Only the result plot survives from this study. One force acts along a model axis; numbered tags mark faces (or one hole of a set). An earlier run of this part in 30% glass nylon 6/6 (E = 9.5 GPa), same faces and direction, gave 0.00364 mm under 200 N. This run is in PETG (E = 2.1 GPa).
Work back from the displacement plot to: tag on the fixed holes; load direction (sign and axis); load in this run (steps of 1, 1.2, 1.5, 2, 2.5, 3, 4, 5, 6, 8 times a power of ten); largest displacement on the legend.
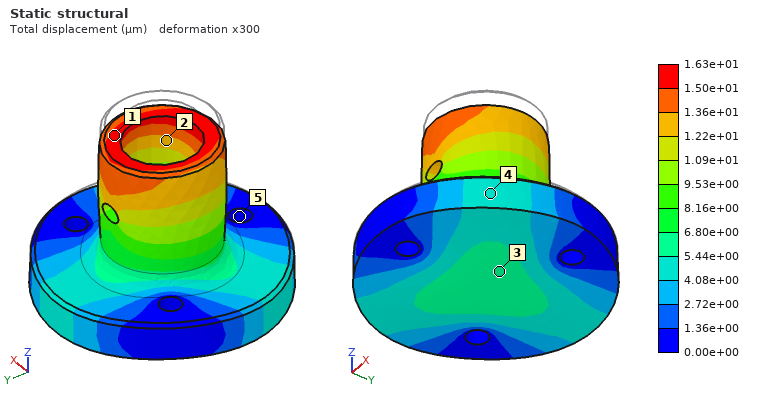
5
-Z
200 N
1.63e+01 µm
